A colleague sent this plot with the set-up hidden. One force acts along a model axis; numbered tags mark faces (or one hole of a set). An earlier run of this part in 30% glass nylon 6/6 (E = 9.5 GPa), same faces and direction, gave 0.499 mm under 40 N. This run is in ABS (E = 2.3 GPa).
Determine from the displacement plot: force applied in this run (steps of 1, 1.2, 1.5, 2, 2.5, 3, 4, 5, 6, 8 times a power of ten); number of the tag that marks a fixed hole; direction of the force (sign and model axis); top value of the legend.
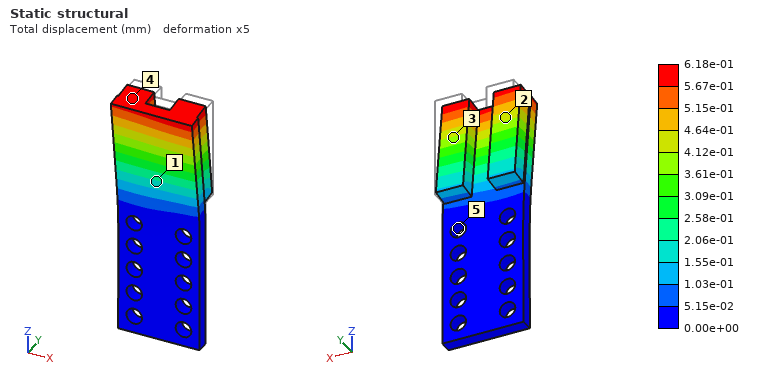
12 N
5
-Y
6.18e-01 mm
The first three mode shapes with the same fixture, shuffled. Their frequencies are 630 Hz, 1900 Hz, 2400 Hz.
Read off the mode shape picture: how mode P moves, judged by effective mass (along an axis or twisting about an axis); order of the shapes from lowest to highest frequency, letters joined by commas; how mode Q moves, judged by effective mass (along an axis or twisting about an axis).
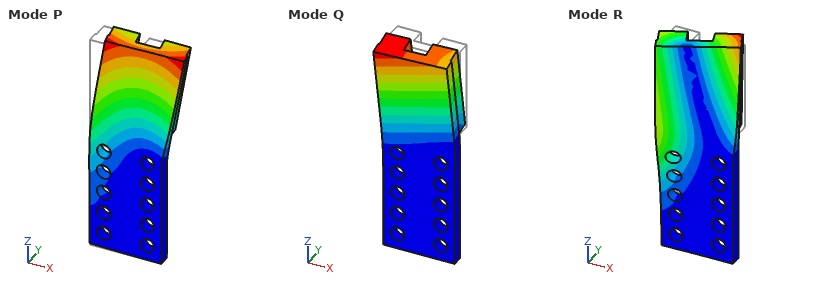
along X
Q, R, P
along Y
